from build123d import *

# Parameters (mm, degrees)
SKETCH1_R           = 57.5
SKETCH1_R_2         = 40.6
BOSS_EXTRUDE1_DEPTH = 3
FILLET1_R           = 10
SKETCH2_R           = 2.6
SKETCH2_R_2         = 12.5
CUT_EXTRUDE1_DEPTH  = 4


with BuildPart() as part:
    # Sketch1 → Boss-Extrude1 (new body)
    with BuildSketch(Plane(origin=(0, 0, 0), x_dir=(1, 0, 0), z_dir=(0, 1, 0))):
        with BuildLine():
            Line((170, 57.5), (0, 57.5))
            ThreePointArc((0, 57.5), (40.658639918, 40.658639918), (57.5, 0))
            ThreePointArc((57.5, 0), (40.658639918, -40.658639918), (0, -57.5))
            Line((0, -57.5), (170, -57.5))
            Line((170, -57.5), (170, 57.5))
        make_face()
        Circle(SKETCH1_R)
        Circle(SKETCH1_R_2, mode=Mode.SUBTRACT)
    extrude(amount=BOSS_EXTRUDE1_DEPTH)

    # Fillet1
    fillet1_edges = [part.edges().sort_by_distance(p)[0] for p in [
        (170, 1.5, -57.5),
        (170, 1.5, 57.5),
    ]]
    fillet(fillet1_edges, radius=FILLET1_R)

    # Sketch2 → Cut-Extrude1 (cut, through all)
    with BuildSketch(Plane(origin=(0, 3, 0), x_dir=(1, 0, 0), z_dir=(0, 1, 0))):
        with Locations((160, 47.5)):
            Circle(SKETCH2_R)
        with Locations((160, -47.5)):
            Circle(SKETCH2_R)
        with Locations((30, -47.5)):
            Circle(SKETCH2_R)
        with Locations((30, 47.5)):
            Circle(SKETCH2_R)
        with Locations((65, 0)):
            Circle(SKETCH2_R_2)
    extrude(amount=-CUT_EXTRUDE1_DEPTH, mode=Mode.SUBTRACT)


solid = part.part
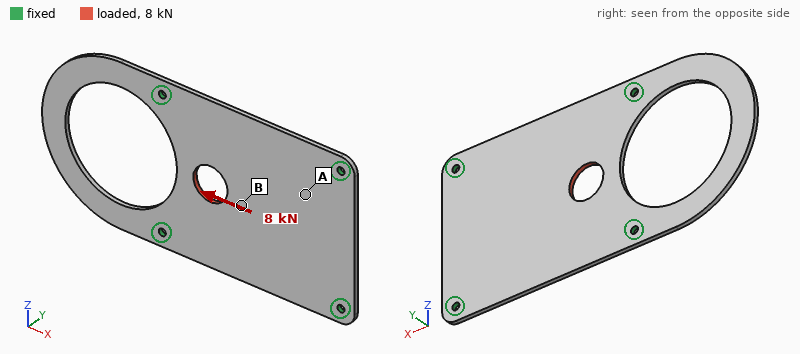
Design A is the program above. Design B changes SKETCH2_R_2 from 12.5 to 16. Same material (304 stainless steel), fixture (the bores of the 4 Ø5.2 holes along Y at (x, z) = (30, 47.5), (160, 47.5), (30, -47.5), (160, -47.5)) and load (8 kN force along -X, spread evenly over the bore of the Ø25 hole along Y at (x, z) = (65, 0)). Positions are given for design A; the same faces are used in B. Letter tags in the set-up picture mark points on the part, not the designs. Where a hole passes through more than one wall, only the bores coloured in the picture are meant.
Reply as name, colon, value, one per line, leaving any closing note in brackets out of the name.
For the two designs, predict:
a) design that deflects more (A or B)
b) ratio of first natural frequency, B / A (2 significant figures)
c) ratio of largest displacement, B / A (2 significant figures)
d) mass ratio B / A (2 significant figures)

design that deflects more: B
ratio of first natural frequency, B / A: 1.00
ratio of largest displacement, B / A: 1.2
mass ratio B / A: 0.98
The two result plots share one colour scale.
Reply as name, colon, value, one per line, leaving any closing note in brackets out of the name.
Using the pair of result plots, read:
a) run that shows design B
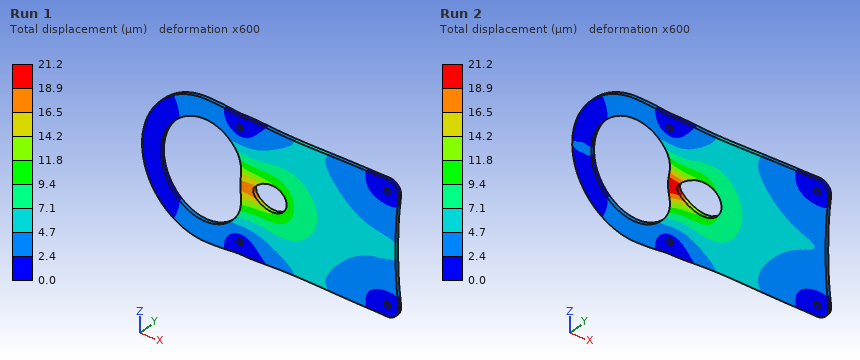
run that shows design B: Run 2
